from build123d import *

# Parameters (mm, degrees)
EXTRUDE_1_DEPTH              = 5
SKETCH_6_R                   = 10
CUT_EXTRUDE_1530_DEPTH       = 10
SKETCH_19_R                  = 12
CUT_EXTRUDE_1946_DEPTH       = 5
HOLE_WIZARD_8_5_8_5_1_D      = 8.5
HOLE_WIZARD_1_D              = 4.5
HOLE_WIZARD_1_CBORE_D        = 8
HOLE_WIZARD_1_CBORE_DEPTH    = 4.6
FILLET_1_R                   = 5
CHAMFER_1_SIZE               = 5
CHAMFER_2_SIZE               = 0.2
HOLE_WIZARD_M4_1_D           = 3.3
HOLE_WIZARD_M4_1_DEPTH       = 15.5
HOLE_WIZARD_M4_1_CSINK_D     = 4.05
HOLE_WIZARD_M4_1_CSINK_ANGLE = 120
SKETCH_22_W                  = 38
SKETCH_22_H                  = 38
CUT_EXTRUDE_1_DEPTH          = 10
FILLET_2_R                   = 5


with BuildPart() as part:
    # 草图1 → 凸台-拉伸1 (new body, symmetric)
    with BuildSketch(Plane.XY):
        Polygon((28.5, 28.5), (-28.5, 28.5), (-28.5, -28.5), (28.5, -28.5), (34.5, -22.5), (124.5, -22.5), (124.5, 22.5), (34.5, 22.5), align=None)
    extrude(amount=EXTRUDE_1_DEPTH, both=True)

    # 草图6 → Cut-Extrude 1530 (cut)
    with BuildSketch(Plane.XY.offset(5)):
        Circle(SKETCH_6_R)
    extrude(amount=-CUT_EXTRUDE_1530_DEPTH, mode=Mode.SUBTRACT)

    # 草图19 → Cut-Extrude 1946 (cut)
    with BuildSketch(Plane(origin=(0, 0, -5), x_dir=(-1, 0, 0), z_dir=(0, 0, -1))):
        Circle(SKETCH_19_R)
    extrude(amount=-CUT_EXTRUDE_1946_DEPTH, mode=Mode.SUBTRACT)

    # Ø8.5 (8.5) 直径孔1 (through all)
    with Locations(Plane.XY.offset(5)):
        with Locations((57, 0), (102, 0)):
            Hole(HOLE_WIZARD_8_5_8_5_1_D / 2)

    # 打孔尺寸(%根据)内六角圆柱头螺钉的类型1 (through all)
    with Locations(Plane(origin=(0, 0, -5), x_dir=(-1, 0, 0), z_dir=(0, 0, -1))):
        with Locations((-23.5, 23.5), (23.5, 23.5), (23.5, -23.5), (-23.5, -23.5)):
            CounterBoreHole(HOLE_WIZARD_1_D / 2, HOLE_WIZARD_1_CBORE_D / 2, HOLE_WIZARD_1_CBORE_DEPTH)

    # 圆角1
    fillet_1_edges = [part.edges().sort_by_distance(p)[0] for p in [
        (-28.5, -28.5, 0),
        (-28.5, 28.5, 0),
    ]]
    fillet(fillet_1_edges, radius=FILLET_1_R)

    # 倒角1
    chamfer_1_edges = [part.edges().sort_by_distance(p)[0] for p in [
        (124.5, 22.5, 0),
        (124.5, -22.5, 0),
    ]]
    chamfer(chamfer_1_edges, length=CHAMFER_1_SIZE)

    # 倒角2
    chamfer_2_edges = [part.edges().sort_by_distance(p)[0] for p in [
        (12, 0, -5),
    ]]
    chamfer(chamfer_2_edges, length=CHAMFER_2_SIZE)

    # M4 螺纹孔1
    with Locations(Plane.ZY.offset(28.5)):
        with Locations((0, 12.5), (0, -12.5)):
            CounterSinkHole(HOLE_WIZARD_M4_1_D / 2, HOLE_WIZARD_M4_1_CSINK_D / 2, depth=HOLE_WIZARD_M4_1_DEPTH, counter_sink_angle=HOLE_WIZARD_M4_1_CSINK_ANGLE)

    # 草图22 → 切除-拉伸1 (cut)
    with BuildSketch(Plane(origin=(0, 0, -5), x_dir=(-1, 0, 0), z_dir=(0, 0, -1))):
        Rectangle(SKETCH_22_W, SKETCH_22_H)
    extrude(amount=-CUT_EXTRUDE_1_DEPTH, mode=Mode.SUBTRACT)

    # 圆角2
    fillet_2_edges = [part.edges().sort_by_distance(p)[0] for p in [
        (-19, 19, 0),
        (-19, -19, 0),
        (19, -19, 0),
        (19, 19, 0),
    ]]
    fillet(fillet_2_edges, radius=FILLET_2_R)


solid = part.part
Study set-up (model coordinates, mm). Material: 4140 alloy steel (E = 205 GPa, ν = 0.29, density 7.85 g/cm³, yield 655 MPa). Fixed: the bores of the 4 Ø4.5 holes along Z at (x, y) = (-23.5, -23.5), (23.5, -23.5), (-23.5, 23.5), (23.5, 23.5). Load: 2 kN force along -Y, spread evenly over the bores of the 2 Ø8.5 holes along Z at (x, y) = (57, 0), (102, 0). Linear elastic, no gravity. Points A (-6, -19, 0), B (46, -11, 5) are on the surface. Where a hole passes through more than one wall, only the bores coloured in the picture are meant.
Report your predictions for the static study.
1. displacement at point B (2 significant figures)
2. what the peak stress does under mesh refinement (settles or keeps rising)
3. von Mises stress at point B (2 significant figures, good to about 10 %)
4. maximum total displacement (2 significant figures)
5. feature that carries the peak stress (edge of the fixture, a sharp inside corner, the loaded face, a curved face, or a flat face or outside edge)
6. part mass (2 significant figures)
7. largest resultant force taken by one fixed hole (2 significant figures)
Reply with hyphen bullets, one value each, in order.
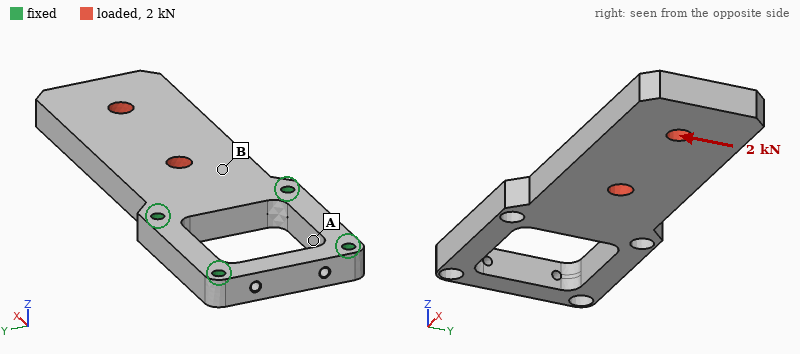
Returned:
- 3.8 µm
- keeps rising
- 14 MPa
- 25 µm
- edge of the fixture
- 460 g
- 2.5 kN
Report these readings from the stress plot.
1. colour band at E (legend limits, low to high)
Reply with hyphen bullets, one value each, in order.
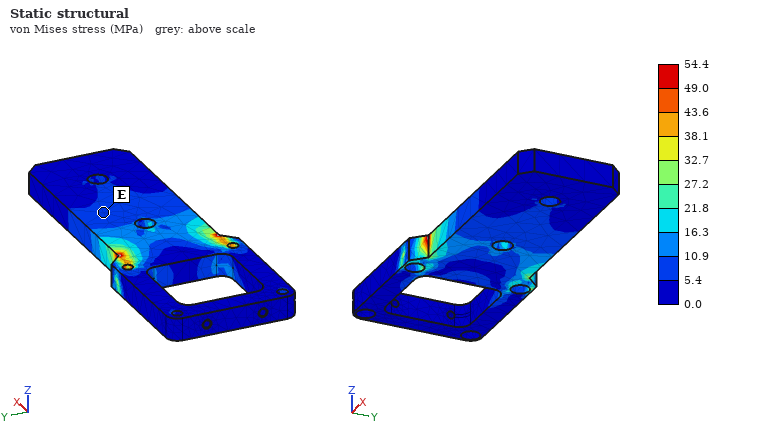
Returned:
- 5.4 to 10.9 MPa
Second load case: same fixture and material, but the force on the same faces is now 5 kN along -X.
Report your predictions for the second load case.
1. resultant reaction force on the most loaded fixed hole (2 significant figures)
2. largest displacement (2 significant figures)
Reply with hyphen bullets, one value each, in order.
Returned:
- 2.4 kN
- 25 µm
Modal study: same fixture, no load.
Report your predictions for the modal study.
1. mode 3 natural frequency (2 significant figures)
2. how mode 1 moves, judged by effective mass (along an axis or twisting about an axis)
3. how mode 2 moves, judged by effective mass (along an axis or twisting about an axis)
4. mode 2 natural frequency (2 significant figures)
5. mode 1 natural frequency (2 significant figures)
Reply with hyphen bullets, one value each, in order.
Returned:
- 3400 Hz
- along Z
- along Y
- 3100 Hz
- 620 Hz
